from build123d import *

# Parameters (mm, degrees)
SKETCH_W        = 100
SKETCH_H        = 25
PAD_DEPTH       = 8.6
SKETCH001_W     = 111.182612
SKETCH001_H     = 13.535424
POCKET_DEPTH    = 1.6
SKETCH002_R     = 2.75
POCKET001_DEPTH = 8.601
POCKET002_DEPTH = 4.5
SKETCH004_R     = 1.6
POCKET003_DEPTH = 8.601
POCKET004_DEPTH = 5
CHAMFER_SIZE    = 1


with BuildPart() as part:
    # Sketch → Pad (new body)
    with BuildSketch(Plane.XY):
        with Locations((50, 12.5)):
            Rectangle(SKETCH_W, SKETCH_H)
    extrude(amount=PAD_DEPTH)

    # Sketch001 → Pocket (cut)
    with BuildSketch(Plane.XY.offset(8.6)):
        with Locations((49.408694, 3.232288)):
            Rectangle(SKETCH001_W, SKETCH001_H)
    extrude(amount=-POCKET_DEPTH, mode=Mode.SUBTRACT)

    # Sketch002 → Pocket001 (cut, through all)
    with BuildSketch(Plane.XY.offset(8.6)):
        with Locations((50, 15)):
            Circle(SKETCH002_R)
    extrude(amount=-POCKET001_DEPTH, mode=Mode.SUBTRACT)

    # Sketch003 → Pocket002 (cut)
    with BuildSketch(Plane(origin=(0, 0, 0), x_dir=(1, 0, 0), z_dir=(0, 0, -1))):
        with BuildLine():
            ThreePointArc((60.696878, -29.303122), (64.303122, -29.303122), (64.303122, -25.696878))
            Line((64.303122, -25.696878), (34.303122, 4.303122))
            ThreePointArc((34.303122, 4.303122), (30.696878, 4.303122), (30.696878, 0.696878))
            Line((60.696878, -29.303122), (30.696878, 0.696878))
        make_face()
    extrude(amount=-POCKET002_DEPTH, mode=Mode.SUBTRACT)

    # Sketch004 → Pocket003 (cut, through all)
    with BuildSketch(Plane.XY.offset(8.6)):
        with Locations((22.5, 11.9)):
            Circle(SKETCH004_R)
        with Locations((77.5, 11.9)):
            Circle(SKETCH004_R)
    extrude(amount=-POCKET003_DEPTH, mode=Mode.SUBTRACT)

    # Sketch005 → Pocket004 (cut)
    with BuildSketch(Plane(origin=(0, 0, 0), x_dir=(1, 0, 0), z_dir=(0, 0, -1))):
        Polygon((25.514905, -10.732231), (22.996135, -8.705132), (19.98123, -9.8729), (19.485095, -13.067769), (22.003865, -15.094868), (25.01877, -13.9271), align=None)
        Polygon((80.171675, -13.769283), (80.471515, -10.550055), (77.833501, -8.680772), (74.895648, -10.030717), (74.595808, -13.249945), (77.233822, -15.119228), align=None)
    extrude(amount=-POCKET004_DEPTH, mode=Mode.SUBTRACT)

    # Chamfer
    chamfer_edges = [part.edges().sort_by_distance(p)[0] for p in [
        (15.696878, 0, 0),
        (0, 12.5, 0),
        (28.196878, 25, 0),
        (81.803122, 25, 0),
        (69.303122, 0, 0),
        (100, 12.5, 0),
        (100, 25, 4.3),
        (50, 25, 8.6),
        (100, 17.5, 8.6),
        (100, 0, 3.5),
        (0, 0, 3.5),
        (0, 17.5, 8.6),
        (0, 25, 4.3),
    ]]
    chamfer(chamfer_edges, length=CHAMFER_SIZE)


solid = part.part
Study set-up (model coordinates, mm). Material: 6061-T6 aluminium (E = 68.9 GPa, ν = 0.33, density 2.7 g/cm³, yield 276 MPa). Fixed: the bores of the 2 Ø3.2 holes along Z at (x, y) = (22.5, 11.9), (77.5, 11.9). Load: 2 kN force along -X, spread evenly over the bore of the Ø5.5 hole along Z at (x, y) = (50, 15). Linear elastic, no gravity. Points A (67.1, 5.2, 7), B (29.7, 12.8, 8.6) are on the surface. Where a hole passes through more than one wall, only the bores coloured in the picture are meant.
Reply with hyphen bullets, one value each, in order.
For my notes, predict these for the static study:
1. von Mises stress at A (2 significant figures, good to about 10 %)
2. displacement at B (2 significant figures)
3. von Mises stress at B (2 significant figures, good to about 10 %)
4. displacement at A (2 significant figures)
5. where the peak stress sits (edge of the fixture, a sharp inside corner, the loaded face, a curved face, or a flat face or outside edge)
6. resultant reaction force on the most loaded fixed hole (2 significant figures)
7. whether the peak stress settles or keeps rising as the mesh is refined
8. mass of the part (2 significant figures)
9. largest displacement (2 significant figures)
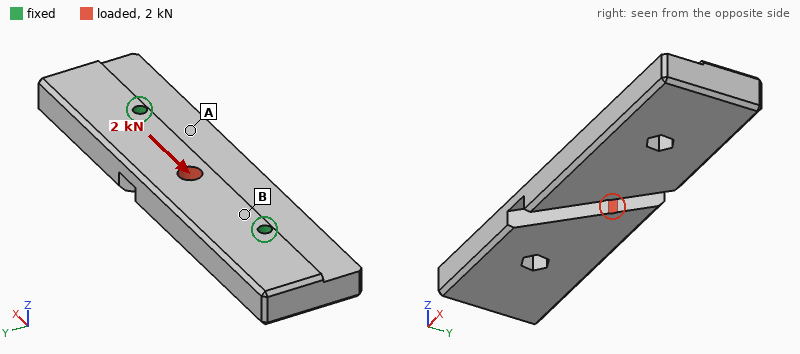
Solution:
- 9.8 MPa
- 2.2 µm
- 19 MPa
- 3.0 µm
- edge of the fixture
- 1.0 kN
- keeps rising
- 50 g
- 8.7 µm
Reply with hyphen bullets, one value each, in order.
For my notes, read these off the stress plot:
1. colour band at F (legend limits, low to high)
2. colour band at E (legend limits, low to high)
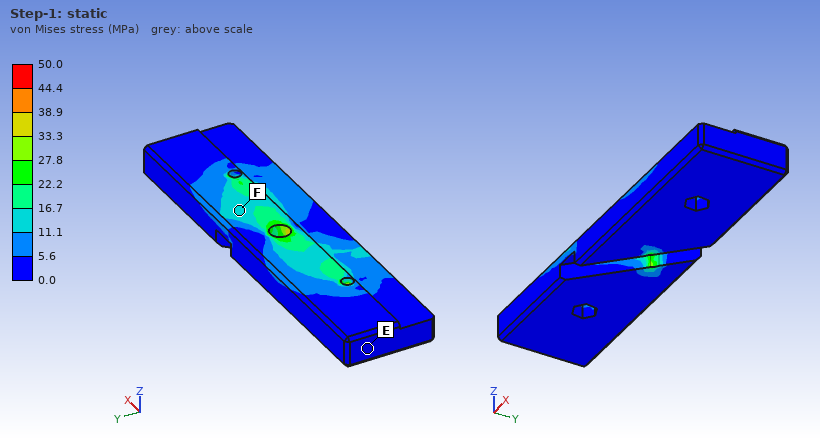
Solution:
- 11.1 to 16.7 MPa
- 0.0 to 5.6 MPa
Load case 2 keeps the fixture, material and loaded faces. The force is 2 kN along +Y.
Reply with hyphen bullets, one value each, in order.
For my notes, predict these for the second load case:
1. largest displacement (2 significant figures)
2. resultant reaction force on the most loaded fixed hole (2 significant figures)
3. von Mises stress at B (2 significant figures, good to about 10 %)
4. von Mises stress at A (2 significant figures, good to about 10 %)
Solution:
- 29 µm
- 1.0 kN
- 20 MPa
- 17 MPa
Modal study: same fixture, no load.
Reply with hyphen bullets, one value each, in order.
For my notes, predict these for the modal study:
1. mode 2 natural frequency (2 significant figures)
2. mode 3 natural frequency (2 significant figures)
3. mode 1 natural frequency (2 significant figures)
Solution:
- 5500 Hz
- 7400 Hz
- 4700 Hz
